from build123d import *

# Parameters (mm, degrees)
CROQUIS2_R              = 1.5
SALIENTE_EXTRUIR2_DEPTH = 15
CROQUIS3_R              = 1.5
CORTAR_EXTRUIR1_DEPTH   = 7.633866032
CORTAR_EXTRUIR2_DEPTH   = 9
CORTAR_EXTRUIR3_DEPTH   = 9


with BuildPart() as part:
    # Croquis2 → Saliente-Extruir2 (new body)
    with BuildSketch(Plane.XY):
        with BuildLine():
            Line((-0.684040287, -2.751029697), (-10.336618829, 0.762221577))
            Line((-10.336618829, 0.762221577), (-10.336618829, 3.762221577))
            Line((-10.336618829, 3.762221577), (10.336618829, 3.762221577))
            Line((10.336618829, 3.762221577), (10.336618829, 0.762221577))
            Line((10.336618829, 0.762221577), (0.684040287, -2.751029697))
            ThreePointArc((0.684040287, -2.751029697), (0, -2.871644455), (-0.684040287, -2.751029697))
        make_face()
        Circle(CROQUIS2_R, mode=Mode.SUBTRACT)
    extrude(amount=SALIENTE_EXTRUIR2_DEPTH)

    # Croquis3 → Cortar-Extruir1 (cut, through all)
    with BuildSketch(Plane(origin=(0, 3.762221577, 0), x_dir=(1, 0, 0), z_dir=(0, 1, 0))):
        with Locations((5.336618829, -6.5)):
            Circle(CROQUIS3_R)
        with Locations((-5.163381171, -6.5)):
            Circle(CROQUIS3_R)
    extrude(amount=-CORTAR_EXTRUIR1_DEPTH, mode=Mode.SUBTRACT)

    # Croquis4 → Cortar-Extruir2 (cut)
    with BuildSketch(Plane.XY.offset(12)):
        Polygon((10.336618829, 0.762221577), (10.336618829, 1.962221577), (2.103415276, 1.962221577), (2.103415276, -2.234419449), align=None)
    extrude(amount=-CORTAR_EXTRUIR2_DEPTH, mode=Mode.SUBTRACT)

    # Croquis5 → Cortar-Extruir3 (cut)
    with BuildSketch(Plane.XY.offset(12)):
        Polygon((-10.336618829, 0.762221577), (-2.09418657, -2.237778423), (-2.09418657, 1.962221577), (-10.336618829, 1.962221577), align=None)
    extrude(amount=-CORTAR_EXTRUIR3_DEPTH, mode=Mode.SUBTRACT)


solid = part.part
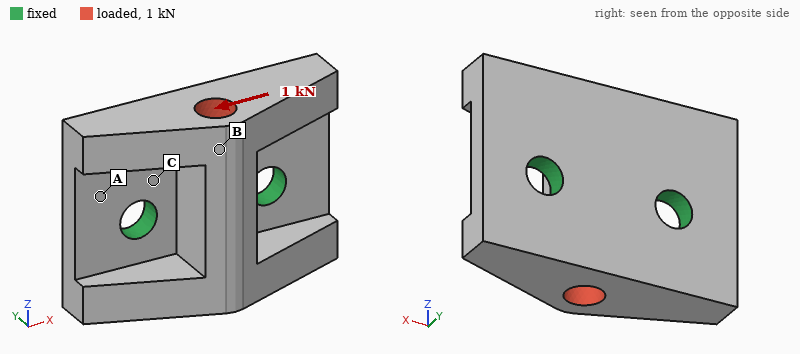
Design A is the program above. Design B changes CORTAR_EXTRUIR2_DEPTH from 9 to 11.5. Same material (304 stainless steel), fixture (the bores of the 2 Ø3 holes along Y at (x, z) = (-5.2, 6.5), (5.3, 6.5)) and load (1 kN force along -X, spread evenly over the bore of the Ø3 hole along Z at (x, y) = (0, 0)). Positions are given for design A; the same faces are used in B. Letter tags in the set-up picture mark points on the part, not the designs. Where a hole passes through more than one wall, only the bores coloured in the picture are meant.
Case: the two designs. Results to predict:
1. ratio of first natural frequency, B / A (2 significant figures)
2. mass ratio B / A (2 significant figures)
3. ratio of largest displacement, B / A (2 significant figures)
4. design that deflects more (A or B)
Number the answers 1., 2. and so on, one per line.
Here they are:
1. 1.0
2. 0.94
3. 1.1
4. B
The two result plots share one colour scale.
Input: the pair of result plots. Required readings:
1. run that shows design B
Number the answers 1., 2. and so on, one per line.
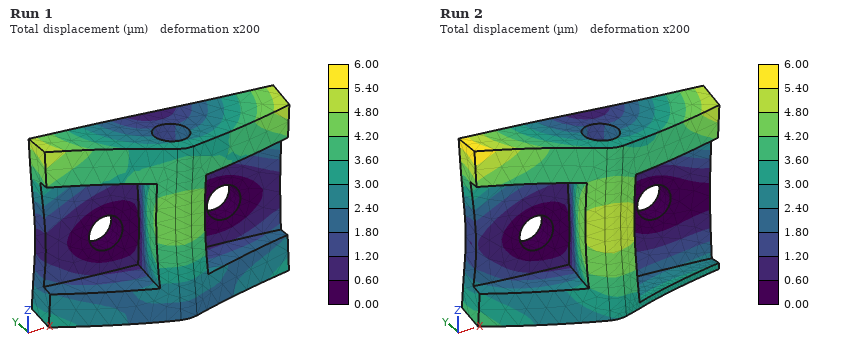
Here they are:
1. Run 2
